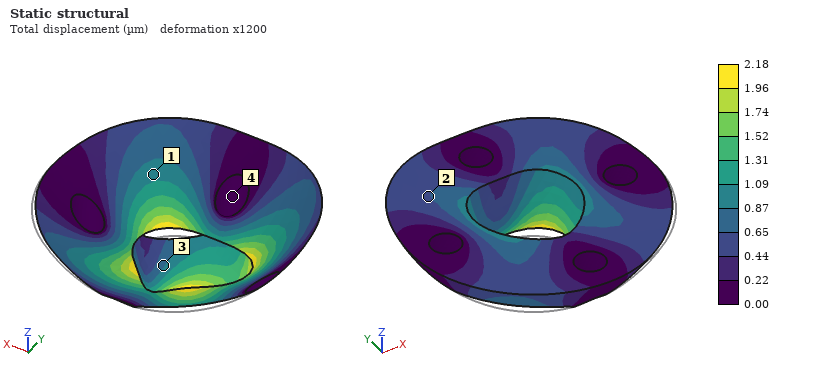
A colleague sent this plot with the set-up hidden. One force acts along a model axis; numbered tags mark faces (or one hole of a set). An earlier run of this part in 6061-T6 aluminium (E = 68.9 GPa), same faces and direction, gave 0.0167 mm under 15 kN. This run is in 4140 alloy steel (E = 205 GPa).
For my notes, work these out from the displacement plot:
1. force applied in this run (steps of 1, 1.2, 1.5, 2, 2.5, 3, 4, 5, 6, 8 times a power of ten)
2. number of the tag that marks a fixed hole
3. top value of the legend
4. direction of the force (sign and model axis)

6 kN
4
2.18 µm
+Y
